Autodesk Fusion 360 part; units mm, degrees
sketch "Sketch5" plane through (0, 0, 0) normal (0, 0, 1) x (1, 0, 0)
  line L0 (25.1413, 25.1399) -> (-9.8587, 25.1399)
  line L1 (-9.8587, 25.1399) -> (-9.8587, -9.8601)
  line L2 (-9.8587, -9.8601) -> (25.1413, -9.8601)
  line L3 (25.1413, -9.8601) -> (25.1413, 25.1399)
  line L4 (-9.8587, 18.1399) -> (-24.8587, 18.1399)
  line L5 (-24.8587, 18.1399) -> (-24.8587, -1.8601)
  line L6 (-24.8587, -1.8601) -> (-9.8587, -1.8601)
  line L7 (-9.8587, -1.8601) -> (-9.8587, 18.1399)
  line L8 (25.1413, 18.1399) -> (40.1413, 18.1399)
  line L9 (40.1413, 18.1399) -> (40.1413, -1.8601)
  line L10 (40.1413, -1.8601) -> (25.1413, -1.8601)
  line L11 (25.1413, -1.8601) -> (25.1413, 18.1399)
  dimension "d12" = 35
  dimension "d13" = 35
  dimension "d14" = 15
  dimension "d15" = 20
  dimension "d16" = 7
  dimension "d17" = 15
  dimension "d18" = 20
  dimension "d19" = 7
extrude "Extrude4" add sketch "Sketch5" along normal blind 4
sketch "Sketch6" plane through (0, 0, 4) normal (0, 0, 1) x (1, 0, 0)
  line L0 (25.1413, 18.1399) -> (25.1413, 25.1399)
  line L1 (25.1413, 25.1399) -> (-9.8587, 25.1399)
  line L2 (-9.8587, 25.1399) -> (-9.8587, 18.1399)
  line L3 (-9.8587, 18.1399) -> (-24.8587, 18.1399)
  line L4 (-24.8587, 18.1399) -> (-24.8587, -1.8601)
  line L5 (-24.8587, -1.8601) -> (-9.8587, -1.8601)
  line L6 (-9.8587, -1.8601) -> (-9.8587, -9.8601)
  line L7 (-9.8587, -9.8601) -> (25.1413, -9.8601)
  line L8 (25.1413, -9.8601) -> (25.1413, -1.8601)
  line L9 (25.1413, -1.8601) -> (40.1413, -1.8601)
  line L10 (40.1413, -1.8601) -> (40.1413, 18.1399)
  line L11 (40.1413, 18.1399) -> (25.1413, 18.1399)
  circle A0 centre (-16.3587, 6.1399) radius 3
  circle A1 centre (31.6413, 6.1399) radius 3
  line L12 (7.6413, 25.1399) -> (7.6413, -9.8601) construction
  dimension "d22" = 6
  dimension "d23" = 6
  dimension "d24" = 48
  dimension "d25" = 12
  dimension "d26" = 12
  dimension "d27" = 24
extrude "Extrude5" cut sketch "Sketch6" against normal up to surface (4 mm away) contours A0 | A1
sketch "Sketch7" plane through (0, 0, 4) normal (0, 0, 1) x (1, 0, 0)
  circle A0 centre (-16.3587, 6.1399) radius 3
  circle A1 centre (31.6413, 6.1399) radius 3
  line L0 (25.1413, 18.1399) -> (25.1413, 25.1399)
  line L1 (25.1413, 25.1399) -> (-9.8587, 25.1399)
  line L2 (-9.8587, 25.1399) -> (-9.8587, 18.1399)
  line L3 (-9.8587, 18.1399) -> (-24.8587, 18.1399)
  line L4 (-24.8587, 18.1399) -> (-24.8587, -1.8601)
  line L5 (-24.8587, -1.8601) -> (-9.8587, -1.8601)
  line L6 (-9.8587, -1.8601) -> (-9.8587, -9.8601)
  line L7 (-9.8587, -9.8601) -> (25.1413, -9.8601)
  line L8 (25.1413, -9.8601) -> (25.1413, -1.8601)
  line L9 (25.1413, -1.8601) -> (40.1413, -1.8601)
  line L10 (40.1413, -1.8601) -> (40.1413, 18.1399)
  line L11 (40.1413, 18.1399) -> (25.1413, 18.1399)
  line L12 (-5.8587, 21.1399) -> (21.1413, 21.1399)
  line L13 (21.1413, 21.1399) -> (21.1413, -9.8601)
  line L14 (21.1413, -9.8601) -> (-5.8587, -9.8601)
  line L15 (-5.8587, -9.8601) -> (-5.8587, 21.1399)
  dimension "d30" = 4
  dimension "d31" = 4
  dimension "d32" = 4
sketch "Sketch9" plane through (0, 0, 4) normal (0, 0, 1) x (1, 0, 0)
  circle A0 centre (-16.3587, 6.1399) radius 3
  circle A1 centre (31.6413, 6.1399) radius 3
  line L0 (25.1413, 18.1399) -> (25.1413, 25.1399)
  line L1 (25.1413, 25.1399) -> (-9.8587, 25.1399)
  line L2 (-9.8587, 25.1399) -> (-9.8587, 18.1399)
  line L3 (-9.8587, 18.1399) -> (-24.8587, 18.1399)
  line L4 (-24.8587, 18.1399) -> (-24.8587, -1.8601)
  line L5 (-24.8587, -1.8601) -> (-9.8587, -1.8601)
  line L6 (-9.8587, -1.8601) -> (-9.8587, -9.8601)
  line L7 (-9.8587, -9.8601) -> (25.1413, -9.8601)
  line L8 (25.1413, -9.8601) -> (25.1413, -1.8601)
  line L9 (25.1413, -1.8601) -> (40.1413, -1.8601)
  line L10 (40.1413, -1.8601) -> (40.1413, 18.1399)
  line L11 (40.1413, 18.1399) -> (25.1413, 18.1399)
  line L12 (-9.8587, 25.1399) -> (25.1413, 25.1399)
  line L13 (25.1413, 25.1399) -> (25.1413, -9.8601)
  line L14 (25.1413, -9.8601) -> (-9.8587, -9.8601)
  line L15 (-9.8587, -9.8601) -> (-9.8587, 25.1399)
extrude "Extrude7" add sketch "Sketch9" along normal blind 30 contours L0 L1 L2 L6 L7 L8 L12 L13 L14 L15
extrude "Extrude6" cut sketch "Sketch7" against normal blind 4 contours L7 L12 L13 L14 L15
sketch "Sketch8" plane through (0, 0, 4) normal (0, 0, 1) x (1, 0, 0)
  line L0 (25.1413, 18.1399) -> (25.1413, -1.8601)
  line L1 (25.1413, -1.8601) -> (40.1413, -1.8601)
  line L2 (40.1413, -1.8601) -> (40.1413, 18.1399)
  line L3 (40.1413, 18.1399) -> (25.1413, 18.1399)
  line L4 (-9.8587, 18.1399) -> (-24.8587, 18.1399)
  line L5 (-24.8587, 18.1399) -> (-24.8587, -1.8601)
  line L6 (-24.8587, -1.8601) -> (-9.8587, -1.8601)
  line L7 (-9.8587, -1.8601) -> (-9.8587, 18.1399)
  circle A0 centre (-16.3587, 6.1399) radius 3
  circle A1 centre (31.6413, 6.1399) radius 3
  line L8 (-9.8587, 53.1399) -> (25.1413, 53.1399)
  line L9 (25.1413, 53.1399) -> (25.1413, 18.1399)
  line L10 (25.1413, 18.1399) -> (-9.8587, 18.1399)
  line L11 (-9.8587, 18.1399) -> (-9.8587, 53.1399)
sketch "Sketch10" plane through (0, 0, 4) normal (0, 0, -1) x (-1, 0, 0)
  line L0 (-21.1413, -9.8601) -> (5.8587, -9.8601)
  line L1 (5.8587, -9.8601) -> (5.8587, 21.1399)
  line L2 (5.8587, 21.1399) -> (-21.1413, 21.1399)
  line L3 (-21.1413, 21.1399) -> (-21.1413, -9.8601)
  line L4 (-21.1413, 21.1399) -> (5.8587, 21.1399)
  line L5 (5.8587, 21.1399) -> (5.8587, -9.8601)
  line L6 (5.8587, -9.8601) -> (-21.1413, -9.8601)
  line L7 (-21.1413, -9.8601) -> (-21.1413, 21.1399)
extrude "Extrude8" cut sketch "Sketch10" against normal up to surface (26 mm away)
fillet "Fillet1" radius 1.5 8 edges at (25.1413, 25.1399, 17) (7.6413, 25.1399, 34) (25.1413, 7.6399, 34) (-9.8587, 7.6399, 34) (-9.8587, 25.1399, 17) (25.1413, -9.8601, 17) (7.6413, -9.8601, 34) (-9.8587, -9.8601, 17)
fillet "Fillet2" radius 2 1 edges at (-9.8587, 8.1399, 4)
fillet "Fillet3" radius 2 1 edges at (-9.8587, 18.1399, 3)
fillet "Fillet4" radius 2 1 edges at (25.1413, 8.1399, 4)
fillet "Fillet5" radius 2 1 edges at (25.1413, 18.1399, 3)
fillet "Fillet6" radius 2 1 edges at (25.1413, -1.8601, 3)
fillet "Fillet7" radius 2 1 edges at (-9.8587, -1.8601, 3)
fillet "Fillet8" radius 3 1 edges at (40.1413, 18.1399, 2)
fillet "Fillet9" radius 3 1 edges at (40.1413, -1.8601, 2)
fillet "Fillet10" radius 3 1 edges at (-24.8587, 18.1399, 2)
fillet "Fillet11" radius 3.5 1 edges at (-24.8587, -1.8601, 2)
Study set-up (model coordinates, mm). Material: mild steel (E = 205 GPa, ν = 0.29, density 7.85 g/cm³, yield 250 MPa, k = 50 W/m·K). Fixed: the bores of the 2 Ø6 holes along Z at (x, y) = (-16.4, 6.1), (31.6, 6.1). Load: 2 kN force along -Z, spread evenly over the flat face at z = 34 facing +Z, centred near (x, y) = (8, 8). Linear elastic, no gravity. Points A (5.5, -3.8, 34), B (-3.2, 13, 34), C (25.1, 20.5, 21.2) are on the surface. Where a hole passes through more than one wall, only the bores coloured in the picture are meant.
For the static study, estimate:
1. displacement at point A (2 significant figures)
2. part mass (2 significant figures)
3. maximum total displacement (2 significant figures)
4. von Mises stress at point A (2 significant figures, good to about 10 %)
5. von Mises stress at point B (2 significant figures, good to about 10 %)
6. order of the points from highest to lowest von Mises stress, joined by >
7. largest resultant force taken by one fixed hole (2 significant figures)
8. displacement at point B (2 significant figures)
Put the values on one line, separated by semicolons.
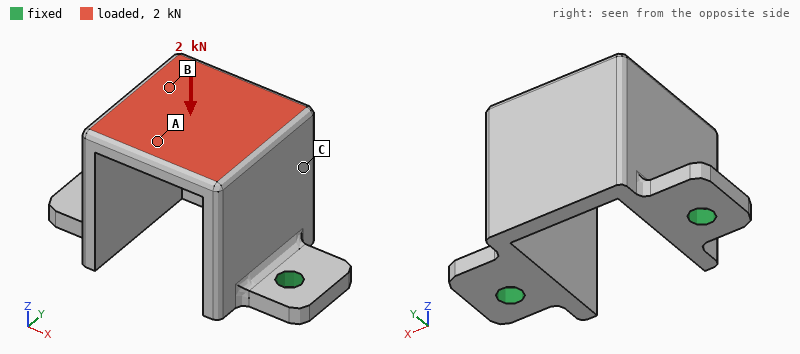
10 µm; 150 g; 11 µm; 30 MPa; 15 MPa; A > B > C; 1.0 kN; 8.4 µm
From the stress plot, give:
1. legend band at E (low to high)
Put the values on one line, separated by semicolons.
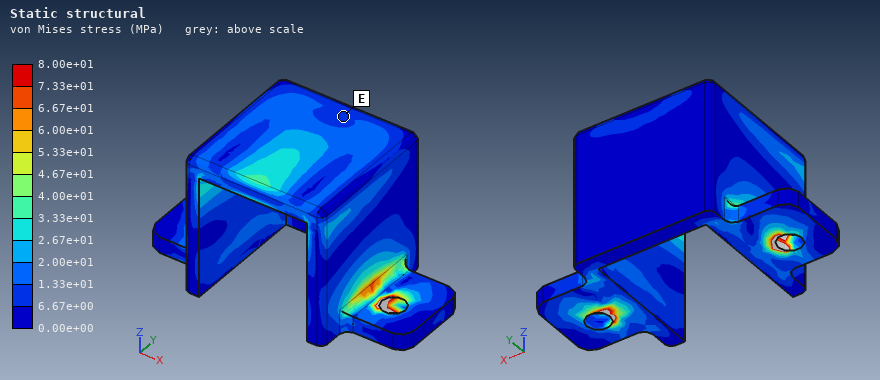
6.67e+00 to 1.33e+01 MPa
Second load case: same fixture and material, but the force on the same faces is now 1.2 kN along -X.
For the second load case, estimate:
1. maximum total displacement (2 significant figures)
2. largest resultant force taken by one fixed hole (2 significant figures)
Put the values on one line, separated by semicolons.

56 µm; 1.0 kN
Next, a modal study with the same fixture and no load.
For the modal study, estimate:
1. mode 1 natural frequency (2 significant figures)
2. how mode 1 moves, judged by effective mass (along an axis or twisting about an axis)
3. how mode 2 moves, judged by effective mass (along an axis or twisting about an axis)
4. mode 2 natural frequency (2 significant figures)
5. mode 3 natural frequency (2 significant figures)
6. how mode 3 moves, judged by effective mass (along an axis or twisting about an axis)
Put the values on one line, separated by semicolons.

2200 Hz; along Y; along X; 3300 Hz; 8300 Hz; along X
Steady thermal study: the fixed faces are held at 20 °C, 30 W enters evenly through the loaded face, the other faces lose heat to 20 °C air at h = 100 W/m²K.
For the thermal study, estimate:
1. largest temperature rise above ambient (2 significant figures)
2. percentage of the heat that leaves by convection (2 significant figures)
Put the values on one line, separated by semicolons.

50 K; 66 %
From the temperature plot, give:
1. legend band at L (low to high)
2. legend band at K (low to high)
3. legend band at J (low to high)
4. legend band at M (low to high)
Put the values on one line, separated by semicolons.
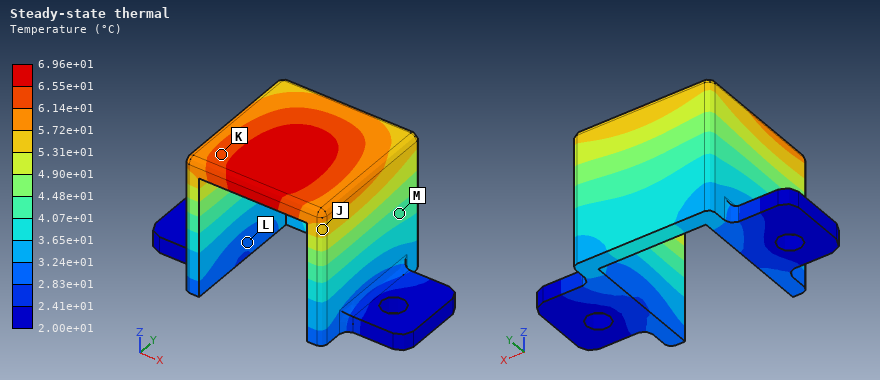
2.83e+01 to 3.24e+01 °C; 6.14e+01 to 6.55e+01 °C; 5.31e+01 to 5.72e+01 °C; 4.07e+01 to 4.48e+01 °C
